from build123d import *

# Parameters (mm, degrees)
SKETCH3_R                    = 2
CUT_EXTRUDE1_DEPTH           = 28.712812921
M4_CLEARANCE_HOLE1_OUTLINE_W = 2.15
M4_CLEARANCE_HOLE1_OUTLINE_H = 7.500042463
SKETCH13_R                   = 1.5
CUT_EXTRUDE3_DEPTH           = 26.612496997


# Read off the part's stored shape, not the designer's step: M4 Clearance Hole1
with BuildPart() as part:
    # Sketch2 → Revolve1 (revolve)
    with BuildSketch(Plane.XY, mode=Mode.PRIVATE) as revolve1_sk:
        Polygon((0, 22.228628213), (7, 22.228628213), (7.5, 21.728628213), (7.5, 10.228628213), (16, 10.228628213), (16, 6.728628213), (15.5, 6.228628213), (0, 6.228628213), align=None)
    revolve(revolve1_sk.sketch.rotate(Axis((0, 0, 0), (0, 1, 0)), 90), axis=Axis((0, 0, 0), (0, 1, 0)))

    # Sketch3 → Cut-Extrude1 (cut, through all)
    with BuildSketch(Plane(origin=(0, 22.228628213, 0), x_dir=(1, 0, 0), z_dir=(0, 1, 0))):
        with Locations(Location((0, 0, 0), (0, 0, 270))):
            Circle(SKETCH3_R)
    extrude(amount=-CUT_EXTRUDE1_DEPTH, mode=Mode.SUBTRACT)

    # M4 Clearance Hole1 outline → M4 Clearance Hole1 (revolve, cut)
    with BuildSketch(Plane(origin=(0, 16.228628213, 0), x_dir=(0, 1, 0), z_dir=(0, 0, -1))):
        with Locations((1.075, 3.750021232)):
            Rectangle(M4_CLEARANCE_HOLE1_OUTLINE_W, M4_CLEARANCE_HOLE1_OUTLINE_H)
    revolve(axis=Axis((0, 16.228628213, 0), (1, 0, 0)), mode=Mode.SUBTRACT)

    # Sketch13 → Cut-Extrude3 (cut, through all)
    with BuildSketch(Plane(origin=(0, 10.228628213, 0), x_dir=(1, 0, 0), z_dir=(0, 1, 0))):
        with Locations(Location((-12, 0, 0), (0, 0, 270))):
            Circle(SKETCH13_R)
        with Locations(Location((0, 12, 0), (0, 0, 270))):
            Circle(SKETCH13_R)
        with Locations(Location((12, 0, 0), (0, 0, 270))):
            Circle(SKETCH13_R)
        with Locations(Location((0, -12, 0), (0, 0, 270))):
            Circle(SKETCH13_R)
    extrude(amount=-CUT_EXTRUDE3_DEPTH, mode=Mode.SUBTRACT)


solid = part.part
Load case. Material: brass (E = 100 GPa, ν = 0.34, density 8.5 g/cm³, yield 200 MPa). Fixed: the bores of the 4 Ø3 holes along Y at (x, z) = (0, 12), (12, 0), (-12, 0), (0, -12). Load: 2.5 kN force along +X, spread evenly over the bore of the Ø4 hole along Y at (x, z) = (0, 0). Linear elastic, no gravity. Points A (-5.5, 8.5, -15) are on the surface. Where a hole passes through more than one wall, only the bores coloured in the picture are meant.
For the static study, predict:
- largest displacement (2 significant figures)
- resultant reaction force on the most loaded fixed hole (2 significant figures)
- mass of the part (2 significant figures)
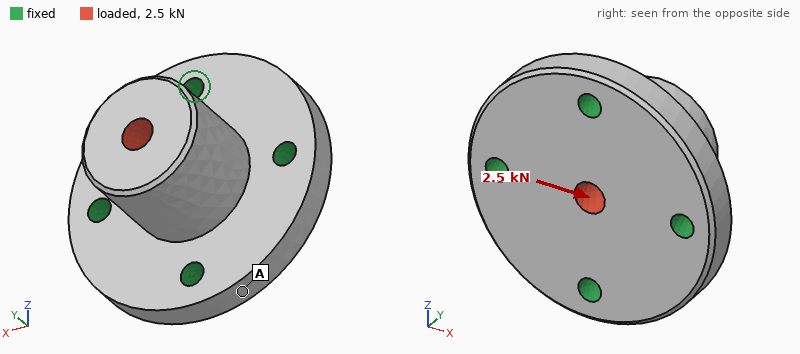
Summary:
13 µm
1.1 kN
42 g
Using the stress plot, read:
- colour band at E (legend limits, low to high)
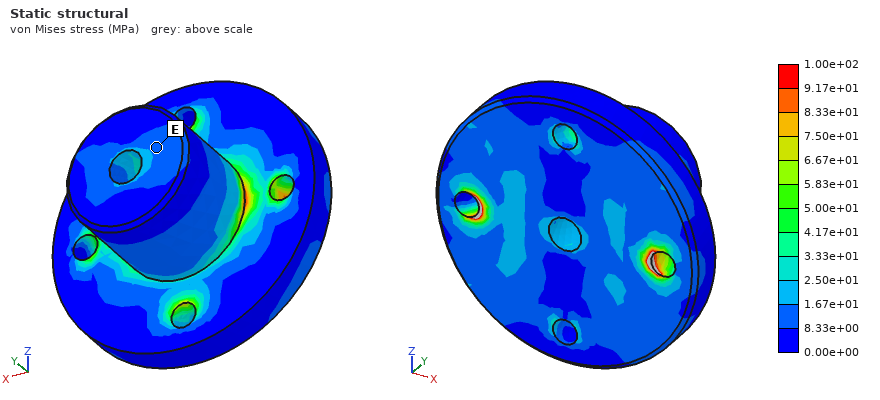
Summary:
8.33e+00 to 1.67e+01 MPa
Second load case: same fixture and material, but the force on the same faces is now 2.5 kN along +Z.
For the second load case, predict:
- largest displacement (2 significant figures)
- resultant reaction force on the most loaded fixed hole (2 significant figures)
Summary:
13 µm
1.1 kN
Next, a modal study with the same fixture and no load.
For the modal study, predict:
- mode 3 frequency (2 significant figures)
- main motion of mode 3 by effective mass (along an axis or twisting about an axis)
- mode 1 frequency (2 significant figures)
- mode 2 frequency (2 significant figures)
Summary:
23 kHz
along Y
17 kHz
17 kHz
